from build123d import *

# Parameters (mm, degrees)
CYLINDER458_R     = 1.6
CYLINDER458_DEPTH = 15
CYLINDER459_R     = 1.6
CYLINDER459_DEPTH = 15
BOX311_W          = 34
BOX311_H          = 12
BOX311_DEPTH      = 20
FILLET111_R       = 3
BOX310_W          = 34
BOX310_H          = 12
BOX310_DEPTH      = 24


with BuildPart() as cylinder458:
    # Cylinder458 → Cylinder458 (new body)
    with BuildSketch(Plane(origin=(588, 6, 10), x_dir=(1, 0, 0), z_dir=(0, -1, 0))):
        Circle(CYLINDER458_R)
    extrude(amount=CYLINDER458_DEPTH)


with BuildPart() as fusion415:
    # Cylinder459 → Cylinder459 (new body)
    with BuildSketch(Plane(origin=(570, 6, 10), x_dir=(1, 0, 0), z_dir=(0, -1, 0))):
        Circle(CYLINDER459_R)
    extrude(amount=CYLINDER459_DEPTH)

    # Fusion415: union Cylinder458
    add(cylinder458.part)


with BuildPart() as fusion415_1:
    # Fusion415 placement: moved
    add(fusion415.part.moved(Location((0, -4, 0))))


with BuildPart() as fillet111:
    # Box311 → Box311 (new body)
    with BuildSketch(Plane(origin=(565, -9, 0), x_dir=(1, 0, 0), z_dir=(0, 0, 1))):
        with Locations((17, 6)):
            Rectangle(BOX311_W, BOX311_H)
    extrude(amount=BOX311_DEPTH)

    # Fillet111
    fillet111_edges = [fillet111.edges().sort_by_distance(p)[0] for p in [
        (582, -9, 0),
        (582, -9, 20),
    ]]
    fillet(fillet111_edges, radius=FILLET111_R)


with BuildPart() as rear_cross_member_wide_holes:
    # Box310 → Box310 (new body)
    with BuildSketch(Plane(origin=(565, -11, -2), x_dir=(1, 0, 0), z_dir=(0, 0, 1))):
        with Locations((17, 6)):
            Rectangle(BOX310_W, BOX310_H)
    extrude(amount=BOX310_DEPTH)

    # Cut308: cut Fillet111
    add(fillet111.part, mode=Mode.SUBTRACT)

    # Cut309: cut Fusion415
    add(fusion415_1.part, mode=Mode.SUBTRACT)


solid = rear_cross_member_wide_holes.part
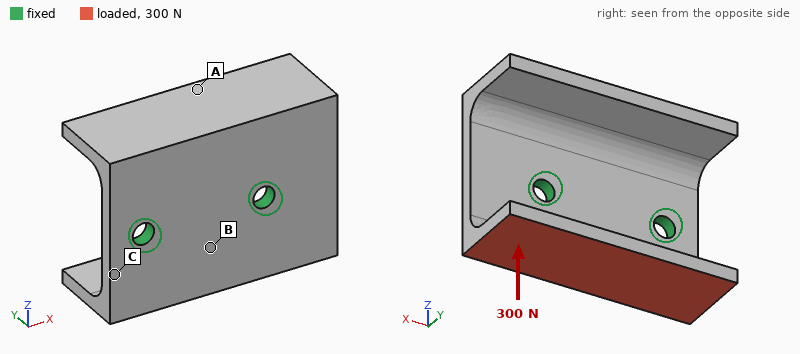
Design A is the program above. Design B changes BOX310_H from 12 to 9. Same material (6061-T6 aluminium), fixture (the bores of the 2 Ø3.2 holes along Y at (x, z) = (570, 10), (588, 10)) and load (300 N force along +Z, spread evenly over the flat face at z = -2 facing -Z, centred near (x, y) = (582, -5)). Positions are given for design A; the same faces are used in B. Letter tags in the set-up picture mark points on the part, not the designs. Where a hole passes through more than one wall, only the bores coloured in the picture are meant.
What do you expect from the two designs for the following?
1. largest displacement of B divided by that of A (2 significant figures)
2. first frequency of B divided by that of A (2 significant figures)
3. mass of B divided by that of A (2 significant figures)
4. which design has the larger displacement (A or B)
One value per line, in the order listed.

35
0.18
0.55
B
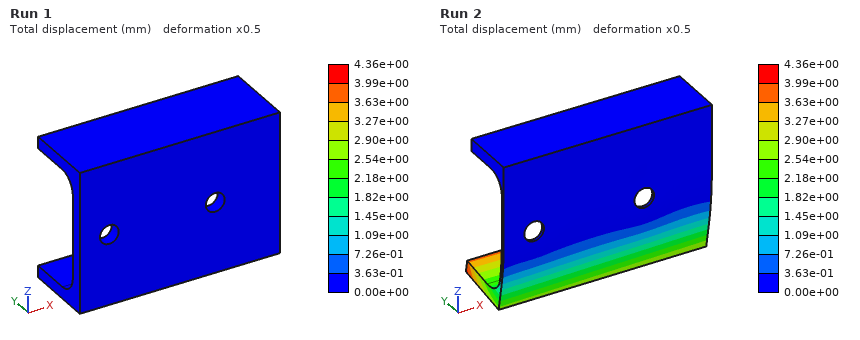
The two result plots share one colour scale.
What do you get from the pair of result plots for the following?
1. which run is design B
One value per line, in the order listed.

Run 2
